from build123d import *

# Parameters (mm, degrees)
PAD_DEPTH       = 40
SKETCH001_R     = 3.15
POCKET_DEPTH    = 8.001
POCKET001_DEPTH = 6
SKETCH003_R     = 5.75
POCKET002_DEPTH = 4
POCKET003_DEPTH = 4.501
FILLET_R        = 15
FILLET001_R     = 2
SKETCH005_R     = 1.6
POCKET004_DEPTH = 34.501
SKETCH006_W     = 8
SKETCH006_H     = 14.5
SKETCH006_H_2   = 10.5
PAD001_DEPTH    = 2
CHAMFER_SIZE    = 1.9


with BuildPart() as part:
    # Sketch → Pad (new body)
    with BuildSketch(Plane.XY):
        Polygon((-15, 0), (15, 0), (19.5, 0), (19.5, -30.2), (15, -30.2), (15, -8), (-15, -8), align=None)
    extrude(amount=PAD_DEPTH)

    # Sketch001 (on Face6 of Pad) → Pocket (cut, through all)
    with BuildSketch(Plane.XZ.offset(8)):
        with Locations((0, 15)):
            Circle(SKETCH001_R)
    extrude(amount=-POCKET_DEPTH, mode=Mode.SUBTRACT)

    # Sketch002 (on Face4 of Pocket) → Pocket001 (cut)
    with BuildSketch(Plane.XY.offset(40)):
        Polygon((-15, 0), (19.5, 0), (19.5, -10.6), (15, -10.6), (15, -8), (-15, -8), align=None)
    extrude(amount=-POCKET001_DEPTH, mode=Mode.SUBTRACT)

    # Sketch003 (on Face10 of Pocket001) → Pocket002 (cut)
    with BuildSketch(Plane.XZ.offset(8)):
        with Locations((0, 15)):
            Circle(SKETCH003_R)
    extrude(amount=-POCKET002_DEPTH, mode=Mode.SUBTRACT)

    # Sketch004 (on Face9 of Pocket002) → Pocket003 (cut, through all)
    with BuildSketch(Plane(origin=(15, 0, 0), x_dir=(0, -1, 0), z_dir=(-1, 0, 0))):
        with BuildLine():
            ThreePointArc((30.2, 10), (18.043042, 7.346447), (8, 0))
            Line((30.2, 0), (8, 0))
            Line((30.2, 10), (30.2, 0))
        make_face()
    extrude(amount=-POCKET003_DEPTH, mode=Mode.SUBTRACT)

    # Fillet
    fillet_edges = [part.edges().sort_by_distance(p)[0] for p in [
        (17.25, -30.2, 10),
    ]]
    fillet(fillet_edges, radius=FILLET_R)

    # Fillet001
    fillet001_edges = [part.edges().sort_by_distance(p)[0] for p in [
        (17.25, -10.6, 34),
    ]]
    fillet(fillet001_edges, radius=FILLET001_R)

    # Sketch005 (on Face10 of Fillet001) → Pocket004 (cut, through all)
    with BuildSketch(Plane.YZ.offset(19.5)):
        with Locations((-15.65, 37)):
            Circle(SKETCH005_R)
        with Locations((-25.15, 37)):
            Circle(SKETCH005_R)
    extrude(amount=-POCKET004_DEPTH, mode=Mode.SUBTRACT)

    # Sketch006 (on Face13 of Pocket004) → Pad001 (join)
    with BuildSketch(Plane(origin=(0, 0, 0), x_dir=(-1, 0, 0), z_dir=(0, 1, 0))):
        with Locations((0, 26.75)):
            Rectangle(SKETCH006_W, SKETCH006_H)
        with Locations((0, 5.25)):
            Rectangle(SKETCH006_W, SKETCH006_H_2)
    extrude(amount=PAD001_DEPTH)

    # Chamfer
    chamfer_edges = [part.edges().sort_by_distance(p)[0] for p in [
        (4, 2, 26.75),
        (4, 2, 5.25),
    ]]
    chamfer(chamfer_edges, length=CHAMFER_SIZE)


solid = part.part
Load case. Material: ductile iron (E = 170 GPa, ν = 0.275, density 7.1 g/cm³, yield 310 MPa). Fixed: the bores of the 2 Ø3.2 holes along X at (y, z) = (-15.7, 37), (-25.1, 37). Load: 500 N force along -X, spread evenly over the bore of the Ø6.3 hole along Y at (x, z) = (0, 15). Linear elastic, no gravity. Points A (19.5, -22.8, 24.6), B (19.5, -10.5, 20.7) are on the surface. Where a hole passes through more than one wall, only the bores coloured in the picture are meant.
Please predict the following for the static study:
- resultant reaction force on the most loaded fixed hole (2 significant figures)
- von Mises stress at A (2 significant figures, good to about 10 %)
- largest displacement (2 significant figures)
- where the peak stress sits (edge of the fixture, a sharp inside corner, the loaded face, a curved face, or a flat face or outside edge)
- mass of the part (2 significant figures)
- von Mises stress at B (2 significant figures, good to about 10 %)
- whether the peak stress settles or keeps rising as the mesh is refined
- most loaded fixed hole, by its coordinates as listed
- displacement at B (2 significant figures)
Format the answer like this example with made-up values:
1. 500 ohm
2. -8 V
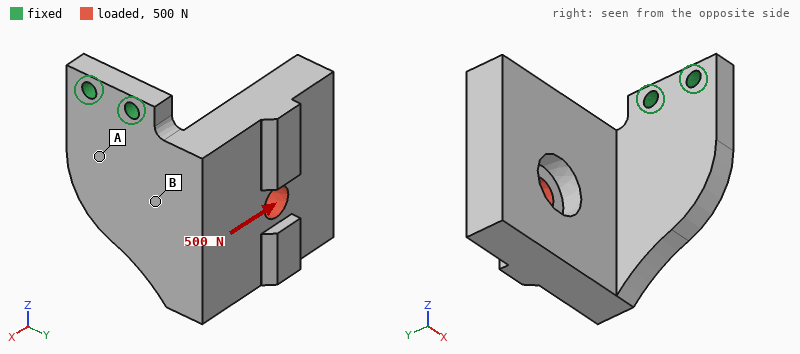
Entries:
1. 810 N
2. 84 MPa
3. 0.25 mm
4. edge of the fixture
5. 87 g
6. 38 MPa
7. keeps rising
8. (-15.7, 37)
9. 0.060 mm
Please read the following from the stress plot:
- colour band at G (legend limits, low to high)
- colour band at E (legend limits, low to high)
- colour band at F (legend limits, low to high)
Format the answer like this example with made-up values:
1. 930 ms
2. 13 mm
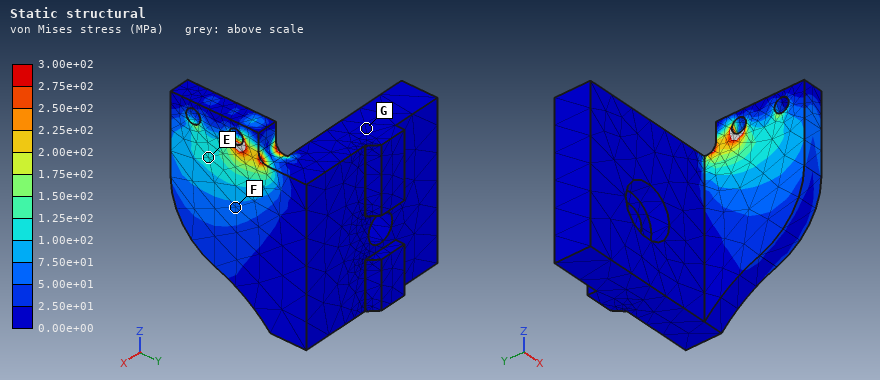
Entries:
1. 0.00e+00 to 2.50e+01 MPa
2. 1.00e+02 to 1.25e+02 MPa
3. 5.00e+01 to 7.50e+01 MPa
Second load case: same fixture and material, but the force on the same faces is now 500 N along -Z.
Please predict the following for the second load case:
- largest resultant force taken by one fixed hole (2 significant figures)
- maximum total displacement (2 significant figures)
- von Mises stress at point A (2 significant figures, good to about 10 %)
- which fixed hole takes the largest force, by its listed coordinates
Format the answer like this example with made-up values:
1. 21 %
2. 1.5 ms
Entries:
1. 1.0 kN
2. 0.19 mm
3. 68 MPa
4. (-15.7, 37)
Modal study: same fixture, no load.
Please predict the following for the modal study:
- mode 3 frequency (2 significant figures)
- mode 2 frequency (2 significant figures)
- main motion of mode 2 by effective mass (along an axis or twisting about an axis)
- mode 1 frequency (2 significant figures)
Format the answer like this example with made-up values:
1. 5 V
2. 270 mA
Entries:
1. 5400 Hz
2. 1600 Hz
3. along Y
4. 990 Hz
